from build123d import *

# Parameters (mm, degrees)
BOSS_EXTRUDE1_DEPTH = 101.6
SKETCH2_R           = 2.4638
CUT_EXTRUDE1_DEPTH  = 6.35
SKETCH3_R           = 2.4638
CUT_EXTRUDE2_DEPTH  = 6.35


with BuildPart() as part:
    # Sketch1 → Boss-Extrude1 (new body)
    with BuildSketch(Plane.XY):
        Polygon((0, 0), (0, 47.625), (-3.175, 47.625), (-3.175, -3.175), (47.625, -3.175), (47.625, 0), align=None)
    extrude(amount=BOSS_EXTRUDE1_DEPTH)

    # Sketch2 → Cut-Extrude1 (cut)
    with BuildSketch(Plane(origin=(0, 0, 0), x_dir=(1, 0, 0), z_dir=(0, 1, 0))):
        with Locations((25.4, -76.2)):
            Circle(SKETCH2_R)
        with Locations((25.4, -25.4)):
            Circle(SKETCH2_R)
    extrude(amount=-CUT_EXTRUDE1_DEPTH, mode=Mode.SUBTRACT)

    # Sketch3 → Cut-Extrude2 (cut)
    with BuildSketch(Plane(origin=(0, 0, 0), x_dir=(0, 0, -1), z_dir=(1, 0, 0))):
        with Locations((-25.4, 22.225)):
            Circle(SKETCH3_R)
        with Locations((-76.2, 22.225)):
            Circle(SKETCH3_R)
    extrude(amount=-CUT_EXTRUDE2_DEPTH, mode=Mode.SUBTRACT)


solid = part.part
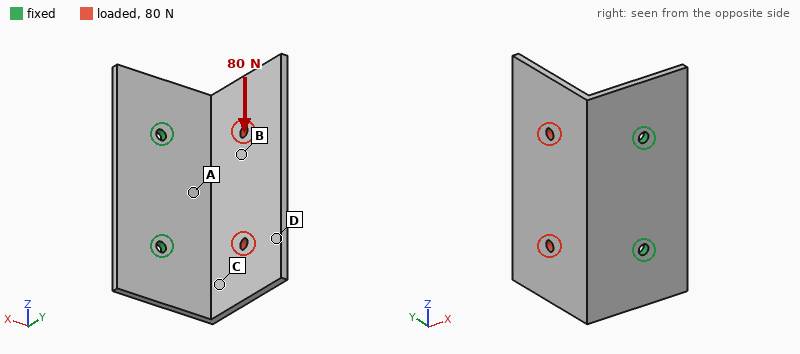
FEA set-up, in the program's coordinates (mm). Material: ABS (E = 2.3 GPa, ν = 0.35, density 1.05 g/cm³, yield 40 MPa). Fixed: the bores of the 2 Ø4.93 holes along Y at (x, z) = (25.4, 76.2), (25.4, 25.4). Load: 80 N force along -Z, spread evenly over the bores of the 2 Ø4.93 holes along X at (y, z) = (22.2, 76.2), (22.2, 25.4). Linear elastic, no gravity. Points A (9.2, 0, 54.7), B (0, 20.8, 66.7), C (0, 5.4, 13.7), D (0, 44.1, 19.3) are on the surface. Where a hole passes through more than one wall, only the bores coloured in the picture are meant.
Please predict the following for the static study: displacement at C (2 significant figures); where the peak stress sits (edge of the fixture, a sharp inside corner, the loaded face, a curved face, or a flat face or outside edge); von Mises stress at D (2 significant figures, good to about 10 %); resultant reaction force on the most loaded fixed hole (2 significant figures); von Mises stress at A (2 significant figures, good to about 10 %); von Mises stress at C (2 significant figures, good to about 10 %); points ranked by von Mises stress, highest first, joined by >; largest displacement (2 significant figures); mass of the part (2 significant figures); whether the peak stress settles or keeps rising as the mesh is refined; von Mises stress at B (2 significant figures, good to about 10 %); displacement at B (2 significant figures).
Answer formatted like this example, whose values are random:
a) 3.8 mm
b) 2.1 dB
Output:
a) 0.58 mm
b) edge of the fixture
c) 0.80 MPa
d) 65 N
e) 4.0 MPa
f) 2.9 MPa
g) A > C > B > D
h) 1.3 mm
i) 33 g
j) keeps rising
k) 1.8 MPa
l) 0.47 mm
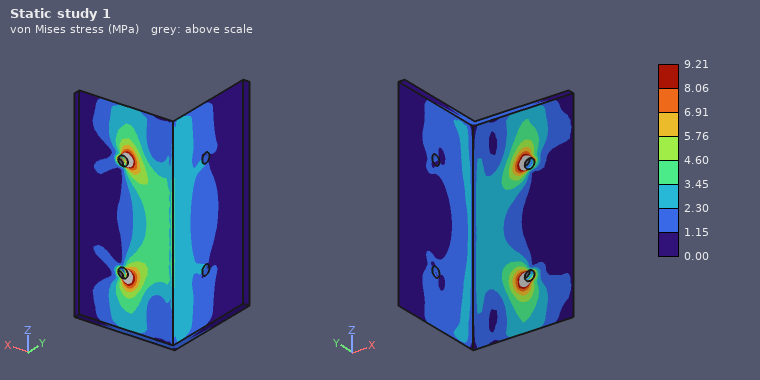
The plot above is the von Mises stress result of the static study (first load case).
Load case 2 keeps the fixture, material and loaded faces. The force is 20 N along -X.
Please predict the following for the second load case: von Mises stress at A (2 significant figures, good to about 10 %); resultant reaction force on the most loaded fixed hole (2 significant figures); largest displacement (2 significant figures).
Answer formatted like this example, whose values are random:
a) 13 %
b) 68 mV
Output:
a) 2.5 MPa
b) 10 N
c) 1.4 mm
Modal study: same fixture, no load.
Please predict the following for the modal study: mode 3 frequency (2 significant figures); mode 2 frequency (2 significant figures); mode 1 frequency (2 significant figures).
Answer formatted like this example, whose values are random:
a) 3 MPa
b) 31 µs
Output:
a) 460 Hz
b) 280 Hz
c) 160 Hz
